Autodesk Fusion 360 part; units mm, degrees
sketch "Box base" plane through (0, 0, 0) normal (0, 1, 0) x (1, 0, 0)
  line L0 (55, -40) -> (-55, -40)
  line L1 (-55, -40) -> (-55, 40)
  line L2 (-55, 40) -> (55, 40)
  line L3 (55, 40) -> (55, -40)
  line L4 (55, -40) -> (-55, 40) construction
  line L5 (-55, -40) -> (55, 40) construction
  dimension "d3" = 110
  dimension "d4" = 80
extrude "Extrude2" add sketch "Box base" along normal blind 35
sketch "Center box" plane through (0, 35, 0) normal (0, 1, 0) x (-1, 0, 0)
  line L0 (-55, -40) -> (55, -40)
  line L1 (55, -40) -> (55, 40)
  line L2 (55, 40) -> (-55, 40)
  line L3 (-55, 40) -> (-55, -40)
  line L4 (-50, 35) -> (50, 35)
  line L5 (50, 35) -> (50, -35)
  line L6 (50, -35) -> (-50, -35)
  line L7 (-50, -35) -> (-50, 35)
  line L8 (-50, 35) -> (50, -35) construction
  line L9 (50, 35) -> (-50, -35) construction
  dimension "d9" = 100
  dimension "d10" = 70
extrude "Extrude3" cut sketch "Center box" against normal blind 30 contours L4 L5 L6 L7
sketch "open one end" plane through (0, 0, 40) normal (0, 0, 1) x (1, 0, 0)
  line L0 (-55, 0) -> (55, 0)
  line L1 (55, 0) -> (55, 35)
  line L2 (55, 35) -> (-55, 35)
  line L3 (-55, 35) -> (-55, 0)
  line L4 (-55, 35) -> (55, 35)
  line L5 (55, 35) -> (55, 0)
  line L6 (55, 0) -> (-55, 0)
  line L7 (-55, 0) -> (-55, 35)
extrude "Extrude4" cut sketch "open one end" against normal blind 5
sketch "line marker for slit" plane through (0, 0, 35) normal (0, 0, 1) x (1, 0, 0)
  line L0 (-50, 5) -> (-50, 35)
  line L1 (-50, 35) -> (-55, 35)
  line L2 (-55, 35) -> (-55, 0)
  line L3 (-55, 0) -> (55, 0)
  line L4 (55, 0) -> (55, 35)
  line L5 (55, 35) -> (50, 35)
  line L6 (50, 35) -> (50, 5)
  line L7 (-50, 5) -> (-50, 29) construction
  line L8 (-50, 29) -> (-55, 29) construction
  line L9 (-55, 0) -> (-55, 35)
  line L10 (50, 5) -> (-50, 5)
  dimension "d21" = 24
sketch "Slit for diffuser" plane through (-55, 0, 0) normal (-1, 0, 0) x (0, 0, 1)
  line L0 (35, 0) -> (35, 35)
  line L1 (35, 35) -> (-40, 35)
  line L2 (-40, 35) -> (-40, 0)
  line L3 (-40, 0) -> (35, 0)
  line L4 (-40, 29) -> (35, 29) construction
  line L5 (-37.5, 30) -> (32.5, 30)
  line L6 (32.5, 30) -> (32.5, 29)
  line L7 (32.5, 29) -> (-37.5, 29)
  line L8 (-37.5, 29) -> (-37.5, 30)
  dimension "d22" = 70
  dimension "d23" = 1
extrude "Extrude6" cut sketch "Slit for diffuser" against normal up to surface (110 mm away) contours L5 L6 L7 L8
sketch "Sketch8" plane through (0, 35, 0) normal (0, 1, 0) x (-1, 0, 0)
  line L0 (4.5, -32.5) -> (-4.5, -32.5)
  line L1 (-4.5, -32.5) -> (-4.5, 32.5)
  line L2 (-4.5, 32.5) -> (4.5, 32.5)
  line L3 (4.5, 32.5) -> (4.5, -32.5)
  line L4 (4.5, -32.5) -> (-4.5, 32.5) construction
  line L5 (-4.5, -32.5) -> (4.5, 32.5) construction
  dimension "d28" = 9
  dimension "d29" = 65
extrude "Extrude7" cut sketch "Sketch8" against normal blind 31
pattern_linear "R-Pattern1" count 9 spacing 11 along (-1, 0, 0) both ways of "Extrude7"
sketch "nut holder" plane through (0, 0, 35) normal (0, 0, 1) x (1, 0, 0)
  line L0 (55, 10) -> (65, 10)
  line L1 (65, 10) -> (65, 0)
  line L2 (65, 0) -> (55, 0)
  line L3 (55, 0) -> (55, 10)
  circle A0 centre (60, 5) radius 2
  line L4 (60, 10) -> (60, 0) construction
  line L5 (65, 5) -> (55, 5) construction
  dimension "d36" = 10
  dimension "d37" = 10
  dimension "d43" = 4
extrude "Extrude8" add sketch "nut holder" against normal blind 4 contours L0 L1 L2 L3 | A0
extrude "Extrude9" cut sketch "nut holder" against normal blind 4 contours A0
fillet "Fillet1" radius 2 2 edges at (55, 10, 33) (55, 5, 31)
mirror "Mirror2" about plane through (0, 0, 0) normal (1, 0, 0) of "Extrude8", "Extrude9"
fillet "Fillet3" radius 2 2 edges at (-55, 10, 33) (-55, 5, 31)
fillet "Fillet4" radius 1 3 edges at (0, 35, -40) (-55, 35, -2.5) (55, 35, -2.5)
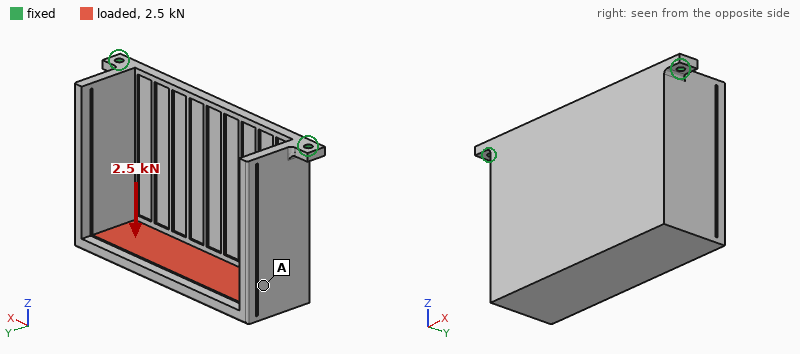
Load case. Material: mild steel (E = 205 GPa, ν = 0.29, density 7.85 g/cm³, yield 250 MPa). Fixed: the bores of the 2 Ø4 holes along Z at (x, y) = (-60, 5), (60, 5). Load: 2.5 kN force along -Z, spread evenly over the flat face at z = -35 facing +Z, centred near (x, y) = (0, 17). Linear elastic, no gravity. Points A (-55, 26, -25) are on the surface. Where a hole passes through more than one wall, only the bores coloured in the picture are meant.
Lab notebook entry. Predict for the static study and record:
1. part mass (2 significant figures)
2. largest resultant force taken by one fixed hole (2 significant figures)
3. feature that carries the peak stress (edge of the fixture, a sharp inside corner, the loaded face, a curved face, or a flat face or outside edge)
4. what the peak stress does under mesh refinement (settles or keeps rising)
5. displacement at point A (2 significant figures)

570 g
1.3 kN
edge of the fixture
keeps rising
0.27 mm
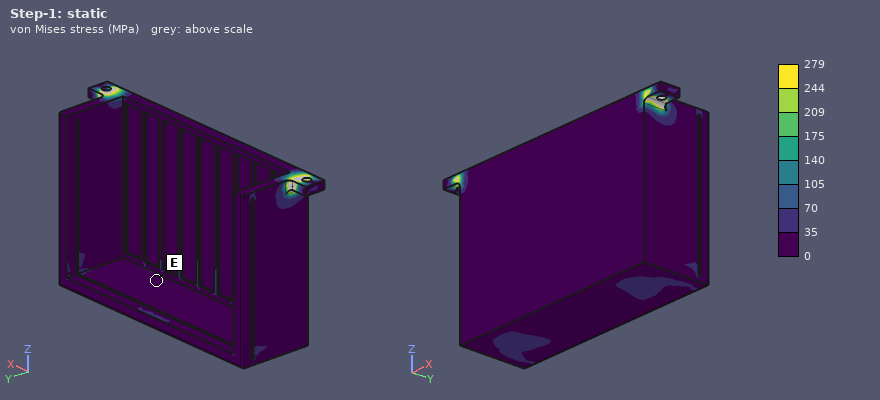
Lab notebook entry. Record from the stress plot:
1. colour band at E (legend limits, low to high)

0 to 35 MPa
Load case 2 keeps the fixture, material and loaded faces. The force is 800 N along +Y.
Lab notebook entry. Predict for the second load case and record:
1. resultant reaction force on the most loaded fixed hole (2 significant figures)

460 N
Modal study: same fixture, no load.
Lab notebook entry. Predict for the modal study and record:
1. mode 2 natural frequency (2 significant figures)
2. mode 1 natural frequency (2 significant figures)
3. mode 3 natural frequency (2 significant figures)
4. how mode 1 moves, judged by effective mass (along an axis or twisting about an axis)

790 Hz
340 Hz
2000 Hz
along Y
